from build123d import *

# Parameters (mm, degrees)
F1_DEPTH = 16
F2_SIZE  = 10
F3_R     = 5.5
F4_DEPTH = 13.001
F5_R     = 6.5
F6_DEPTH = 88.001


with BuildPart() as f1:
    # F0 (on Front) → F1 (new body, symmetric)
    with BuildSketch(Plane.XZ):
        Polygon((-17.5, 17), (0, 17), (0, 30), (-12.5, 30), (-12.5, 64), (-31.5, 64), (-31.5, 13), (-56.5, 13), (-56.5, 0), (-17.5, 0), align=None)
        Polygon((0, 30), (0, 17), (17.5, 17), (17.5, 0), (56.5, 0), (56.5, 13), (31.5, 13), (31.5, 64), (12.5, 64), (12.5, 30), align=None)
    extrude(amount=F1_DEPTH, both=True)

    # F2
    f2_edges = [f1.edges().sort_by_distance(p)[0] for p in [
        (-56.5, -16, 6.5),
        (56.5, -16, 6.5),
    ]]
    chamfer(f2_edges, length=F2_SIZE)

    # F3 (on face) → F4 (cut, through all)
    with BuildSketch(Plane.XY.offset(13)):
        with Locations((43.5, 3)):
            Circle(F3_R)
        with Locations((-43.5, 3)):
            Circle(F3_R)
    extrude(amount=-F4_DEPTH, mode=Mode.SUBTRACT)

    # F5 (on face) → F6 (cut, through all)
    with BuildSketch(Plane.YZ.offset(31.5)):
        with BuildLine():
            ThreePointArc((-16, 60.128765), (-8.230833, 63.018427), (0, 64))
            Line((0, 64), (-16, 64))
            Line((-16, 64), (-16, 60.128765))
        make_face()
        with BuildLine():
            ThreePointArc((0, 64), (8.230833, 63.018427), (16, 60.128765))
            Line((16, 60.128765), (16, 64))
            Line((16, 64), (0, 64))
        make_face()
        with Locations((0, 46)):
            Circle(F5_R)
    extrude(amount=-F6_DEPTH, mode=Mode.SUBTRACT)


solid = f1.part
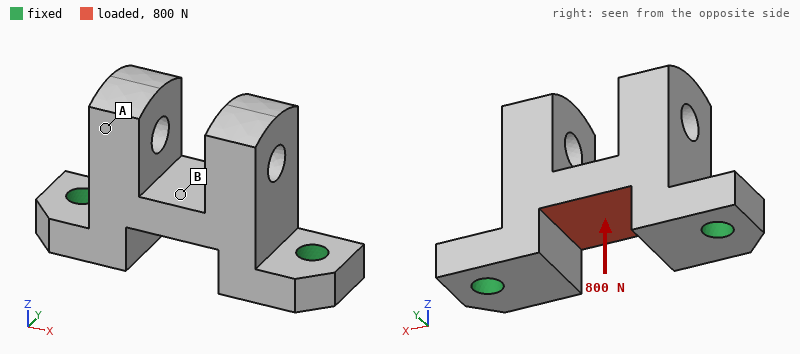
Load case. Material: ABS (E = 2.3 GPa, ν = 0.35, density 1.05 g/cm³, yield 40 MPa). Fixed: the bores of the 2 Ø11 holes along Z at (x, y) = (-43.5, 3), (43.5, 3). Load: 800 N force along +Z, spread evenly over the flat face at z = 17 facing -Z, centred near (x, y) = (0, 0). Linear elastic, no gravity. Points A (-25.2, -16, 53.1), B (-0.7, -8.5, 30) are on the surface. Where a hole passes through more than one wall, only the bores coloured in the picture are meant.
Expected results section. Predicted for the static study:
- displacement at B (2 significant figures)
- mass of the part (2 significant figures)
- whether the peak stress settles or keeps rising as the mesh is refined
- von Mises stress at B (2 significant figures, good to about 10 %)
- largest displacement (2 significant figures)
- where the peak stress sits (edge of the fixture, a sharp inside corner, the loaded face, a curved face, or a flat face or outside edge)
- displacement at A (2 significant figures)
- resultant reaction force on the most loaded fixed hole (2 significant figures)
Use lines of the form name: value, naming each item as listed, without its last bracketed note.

displacement at B: 0.089 mm
mass of the part: 98 g
whether the peak stress settles or keeps rising as the mesh is refined: keeps rising
von Mises stress at B: 3.7 MPa
largest displacement: 0.12 mm
where the peak stress sits: edge of the fixture
displacement at A: 0.087 mm
resultant reaction force on the most loaded fixed hole: 570 N
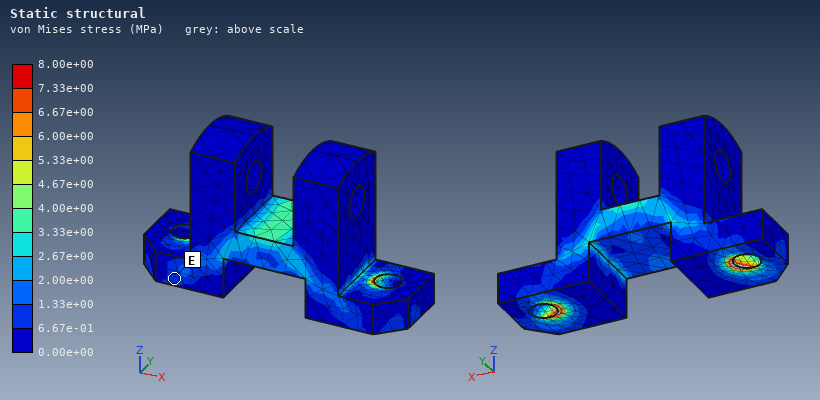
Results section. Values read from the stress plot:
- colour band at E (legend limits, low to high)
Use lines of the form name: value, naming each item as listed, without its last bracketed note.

colour band at E: 6.67e-01 to 1.33e+00 MPa
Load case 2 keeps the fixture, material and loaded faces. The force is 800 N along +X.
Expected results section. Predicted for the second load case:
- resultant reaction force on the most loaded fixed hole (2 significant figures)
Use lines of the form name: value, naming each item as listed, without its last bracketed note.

resultant reaction force on the most loaded fixed hole: 410 N
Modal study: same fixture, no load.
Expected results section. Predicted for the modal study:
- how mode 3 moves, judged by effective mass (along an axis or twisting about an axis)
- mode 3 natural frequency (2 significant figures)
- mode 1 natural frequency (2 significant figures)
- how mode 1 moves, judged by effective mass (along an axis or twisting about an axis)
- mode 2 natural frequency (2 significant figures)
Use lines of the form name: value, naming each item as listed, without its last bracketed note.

how mode 3 moves, judged by effective mass: along X
mode 3 natural frequency: 1700 Hz
mode 1 natural frequency: 820 Hz
how mode 1 moves, judged by effective mass: along Y
mode 2 natural frequency: 1300 Hz
